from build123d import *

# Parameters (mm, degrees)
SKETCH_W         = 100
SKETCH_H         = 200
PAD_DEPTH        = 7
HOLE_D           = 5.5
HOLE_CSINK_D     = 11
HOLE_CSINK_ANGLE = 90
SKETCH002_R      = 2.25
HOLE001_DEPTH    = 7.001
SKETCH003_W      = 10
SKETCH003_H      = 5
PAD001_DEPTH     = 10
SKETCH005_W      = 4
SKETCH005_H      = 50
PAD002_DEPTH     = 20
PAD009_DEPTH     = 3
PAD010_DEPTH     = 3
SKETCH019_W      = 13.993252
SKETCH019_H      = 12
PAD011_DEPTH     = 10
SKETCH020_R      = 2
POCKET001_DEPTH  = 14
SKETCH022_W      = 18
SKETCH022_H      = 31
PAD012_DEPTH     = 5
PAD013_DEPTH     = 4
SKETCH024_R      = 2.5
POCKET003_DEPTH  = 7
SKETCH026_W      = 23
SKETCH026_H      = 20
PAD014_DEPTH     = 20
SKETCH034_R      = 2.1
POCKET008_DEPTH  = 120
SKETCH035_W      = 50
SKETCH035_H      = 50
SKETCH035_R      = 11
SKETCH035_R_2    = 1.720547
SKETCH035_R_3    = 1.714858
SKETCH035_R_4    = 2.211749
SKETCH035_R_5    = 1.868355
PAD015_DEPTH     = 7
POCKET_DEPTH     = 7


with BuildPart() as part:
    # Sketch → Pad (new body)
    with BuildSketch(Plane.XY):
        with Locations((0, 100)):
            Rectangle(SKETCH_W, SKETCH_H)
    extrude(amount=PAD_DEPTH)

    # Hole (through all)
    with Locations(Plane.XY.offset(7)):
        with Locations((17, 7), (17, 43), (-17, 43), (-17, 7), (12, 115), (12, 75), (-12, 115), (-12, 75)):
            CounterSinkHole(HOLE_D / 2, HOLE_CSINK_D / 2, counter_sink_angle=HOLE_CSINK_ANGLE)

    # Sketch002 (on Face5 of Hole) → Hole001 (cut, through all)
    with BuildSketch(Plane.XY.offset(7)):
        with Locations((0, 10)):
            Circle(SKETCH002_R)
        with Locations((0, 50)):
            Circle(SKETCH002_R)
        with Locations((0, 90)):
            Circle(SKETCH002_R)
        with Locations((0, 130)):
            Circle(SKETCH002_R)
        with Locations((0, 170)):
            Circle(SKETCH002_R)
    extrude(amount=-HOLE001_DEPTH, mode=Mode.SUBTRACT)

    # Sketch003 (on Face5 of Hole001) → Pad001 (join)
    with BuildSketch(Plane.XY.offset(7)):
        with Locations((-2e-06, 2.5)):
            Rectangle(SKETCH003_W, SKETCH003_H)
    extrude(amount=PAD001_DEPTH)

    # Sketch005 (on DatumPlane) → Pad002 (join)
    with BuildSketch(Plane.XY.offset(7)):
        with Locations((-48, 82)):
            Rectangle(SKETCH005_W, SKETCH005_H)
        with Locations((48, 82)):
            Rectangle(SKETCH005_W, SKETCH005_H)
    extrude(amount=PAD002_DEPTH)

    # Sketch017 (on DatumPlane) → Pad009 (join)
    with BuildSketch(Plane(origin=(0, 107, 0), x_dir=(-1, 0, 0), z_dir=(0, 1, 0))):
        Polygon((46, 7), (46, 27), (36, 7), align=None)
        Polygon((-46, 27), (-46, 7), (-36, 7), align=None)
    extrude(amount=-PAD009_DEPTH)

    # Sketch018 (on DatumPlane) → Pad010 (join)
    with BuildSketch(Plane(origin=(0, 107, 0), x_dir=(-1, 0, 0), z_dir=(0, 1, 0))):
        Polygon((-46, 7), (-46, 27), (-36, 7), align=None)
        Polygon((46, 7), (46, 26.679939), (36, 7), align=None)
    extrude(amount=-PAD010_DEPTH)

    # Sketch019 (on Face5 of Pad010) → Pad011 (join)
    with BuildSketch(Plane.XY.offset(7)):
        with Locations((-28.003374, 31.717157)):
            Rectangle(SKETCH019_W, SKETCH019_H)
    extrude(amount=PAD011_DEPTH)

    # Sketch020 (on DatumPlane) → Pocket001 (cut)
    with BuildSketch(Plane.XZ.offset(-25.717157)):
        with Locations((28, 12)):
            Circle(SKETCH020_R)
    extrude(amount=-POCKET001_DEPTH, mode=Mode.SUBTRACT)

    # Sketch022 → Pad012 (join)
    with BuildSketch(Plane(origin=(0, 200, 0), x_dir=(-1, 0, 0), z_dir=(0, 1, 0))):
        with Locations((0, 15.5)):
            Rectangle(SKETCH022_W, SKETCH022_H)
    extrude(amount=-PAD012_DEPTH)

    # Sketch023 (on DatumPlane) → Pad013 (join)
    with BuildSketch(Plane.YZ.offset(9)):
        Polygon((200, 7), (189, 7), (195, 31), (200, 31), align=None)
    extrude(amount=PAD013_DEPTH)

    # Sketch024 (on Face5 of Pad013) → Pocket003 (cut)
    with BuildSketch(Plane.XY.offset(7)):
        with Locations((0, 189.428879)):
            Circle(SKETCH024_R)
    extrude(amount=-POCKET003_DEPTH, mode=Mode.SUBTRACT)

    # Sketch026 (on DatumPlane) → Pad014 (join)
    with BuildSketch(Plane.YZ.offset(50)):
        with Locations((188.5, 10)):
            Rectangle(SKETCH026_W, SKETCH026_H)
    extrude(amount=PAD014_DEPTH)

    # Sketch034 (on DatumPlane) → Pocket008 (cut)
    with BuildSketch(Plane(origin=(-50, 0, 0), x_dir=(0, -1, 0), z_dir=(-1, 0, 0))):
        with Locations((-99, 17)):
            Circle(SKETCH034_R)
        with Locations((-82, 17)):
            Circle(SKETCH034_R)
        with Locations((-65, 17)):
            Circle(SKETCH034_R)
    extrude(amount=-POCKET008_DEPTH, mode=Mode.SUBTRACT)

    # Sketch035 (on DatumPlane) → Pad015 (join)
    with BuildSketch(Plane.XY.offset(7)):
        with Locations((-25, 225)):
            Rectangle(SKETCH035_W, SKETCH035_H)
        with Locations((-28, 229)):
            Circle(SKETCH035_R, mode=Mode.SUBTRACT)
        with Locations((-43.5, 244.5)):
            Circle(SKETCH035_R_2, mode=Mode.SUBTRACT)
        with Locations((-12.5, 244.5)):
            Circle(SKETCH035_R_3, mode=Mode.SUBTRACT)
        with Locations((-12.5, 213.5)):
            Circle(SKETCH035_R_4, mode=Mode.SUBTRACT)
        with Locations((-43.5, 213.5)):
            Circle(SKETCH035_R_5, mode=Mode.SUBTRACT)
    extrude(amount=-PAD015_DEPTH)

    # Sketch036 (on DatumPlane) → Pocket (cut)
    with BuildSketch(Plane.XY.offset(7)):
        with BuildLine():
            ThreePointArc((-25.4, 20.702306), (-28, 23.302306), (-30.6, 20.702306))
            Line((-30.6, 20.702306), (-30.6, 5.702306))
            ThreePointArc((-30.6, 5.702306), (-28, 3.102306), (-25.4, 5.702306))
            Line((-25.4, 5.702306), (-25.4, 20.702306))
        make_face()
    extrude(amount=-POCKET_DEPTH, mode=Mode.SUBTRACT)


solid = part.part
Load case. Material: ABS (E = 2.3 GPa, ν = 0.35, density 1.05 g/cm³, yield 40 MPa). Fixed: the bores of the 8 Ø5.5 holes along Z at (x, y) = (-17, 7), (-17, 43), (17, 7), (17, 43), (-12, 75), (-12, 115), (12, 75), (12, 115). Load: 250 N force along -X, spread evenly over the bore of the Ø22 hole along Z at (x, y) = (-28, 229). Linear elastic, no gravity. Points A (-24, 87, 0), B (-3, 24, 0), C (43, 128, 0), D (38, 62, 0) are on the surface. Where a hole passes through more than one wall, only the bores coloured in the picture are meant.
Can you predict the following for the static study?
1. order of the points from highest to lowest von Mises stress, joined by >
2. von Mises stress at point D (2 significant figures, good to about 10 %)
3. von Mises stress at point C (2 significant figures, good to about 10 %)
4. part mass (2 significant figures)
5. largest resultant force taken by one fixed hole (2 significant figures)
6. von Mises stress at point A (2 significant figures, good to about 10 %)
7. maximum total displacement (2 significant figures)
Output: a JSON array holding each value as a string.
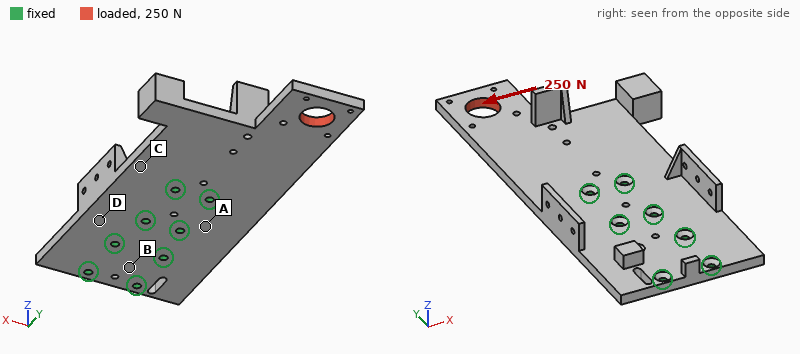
["C > A > D > B", "0.64 MPa", "1.6 MPa", "180 g", "350 N", "1.2 MPa", "0.47 mm"]
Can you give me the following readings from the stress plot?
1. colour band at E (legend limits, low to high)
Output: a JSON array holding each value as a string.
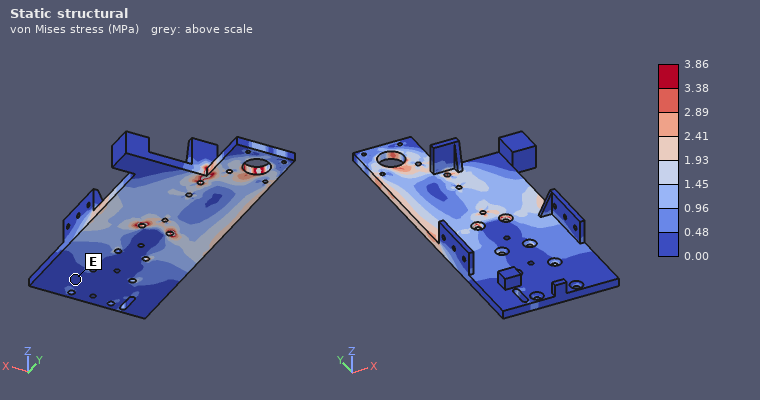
["0.00 to 0.48 MPa"]
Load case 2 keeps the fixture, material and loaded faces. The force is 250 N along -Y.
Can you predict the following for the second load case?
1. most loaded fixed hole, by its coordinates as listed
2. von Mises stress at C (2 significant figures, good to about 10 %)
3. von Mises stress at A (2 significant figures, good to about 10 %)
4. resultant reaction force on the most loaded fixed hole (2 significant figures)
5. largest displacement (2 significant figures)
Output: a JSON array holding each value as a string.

["(-12, 115)", "0.25 MPa", "0.45 MPa", "150 N", "0.11 mm"]
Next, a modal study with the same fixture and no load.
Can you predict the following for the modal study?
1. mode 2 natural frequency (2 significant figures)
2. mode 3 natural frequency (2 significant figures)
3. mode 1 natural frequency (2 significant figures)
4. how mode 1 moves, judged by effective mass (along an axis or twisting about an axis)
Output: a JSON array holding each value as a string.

["210 Hz", "510 Hz", "110 Hz", "along Z"]
